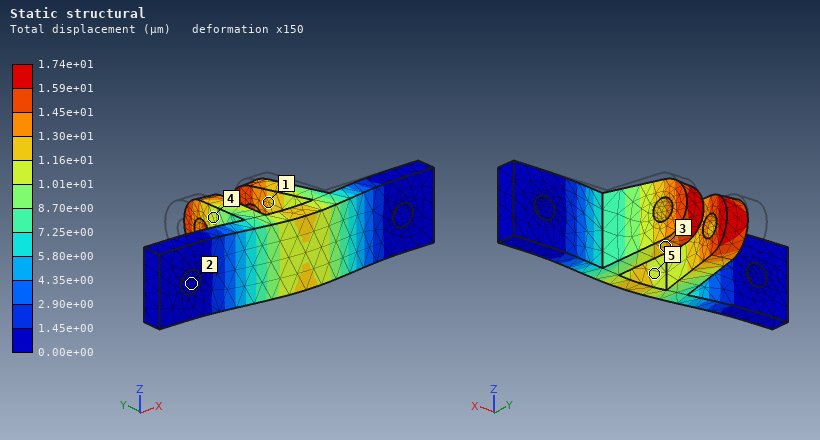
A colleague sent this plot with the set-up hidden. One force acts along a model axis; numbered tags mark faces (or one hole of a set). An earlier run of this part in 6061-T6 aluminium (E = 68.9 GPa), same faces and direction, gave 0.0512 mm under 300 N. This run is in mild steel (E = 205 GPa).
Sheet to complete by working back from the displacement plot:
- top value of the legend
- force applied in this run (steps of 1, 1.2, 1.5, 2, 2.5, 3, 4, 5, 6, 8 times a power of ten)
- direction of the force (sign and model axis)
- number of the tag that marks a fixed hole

1.74e+01 µm
300 N
-Y
2
